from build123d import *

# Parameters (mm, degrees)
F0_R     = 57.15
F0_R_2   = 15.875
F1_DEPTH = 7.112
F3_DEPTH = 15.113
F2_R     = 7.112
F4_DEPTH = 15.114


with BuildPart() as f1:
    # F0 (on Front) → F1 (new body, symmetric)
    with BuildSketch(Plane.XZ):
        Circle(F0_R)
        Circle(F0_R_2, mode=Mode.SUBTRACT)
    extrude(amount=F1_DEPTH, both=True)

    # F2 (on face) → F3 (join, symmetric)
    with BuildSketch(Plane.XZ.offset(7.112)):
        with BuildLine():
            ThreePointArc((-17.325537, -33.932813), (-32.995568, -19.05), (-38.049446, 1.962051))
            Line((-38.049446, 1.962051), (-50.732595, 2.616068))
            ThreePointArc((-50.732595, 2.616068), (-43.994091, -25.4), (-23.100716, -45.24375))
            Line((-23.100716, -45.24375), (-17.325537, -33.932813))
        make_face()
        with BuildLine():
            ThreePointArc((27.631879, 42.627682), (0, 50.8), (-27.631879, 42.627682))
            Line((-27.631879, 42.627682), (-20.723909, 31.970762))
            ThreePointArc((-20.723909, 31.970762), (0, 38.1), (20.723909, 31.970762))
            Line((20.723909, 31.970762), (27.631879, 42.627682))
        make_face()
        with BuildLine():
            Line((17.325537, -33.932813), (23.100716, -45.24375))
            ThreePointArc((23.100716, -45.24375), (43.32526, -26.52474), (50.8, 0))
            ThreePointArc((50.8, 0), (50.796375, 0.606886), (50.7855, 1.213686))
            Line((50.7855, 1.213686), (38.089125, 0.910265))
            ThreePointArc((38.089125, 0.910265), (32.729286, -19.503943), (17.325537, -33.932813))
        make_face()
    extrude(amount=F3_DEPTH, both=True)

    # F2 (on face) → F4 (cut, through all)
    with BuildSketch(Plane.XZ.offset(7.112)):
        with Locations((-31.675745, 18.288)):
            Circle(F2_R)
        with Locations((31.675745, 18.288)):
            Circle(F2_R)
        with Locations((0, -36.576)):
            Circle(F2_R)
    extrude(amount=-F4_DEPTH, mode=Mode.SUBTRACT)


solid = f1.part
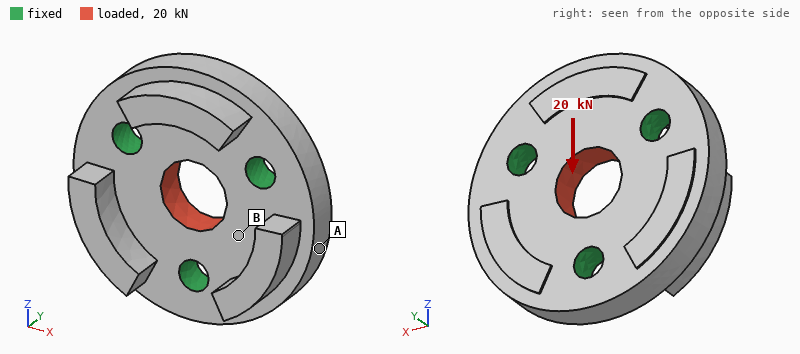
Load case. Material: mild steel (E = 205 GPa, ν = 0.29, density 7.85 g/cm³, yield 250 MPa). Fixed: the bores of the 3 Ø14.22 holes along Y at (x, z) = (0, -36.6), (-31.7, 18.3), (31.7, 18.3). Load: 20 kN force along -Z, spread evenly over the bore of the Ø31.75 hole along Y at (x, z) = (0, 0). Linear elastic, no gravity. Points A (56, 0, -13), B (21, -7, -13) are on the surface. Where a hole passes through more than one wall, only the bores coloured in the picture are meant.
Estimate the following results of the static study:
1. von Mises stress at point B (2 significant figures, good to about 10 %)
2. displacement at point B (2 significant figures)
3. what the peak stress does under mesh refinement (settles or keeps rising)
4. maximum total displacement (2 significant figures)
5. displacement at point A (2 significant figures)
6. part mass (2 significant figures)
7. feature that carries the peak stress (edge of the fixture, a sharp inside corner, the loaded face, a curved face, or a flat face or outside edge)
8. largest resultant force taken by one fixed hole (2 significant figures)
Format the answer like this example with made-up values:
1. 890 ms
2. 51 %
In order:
1. 7.9 MPa
2. 1.3 µm
3. keeps rising
4. 2.8 µm
5. 0.47 µm
6. 1.2 kg
7. edge of the fixture
8. 6.8 kN
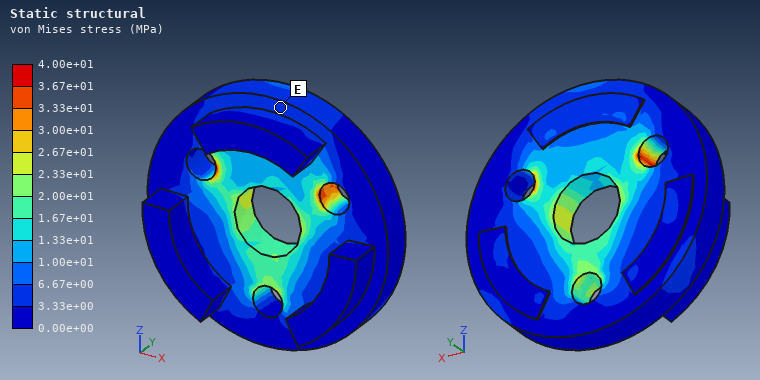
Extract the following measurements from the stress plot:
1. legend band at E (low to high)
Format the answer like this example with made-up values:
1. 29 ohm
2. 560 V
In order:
1. 3.33e+00 to 6.67e+00 MPa
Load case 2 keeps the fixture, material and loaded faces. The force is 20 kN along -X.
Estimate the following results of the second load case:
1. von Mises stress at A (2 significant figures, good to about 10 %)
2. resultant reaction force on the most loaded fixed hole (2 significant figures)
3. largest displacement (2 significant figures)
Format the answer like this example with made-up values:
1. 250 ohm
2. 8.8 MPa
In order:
1. 5.3 MPa
2. 6.9 kN
3. 2.6 µm
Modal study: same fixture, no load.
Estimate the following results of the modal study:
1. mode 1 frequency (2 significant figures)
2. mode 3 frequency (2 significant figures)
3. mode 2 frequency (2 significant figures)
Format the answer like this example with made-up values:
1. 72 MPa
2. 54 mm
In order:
1. 6900 Hz
2. 7200 Hz
3. 6900 Hz
